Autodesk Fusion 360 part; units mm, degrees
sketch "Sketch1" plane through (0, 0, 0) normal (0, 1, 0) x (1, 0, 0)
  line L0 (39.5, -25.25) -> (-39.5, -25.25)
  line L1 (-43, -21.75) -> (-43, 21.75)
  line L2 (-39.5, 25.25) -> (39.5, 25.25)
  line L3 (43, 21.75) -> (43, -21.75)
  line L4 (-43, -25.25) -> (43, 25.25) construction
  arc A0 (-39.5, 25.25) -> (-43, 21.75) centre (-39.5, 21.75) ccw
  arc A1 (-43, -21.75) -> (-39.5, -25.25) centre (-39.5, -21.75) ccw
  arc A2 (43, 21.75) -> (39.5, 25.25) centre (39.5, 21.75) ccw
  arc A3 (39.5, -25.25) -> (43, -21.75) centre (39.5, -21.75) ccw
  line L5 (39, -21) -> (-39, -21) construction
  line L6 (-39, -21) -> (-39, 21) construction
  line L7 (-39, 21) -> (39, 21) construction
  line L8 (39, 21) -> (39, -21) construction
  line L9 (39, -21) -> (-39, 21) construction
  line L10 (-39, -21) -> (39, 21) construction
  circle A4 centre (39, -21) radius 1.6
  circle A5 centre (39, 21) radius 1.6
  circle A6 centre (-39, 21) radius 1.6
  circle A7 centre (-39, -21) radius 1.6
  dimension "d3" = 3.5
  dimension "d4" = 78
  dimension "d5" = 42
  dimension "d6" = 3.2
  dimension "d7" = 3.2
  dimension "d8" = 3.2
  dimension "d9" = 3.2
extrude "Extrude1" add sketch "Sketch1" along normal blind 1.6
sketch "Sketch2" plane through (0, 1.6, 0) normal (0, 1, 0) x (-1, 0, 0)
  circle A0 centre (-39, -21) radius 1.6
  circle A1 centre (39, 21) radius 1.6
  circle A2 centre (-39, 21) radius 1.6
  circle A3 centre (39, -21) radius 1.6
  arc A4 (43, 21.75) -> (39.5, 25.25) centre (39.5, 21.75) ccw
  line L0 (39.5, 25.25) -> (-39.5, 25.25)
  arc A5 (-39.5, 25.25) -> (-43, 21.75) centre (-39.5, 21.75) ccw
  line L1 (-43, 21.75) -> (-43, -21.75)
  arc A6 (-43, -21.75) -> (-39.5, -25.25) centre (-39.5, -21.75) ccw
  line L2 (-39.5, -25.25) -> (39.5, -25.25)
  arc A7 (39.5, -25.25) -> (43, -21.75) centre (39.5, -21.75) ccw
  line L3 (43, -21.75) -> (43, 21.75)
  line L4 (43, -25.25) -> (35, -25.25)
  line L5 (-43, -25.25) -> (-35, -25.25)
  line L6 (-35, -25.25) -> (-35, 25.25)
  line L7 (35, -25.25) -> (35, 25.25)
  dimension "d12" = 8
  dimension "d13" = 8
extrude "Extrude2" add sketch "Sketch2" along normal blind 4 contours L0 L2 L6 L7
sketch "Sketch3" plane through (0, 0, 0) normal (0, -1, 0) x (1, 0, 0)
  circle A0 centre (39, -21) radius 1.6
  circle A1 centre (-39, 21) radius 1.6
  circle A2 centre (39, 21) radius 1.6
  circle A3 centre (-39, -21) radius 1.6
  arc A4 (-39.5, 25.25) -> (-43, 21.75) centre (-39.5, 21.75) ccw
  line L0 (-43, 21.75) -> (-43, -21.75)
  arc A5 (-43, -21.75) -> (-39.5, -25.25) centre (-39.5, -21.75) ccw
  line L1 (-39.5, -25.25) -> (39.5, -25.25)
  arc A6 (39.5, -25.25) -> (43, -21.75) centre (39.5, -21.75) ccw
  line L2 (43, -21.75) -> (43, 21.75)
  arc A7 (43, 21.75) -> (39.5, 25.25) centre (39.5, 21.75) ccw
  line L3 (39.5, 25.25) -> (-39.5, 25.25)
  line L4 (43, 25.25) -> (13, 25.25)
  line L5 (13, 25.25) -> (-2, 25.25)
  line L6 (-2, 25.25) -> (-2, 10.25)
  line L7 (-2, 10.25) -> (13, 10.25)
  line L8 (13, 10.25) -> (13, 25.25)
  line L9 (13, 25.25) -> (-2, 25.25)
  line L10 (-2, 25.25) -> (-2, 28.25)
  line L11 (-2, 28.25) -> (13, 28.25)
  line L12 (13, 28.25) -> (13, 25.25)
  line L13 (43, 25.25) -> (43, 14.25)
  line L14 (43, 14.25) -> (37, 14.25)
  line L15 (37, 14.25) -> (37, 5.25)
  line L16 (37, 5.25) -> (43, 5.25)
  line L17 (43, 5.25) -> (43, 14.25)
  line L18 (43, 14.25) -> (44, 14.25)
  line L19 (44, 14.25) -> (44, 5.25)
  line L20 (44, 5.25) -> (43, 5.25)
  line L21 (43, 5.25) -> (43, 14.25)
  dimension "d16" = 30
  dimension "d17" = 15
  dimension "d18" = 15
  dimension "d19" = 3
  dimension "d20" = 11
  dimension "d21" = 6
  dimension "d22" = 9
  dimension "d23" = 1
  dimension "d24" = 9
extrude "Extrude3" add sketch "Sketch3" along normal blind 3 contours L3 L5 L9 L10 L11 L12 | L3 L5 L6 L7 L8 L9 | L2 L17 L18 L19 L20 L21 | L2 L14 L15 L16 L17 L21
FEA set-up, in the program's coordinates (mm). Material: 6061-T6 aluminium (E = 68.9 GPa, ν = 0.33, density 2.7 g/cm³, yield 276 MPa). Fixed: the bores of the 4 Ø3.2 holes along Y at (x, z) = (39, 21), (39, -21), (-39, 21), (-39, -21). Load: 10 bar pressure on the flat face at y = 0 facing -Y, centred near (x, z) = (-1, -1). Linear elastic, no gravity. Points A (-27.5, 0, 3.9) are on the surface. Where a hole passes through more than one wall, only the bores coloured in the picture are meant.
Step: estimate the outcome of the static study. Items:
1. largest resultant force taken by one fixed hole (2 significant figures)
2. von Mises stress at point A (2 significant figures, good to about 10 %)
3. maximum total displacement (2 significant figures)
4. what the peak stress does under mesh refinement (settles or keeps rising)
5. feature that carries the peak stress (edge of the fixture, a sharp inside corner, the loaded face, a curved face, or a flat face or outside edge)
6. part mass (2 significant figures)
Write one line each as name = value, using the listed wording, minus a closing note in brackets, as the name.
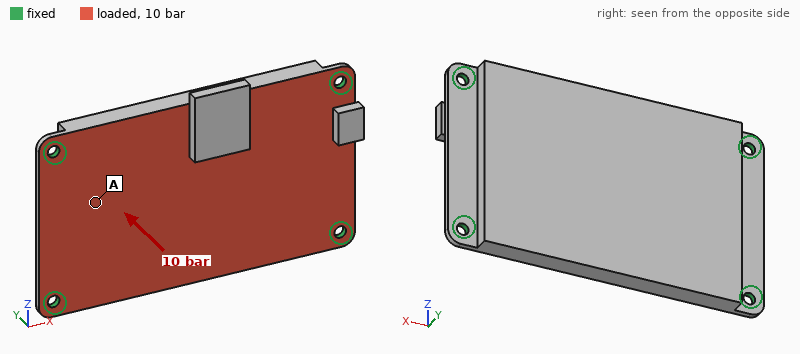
largest resultant force taken by one fixed hole = 2.3 kN
von Mises stress at point A = 28 MPa
maximum total displacement = 0.26 mm
what the peak stress does under mesh refinement = keeps rising
feature that carries the peak stress = edge of the fixture
part mass = 59 g
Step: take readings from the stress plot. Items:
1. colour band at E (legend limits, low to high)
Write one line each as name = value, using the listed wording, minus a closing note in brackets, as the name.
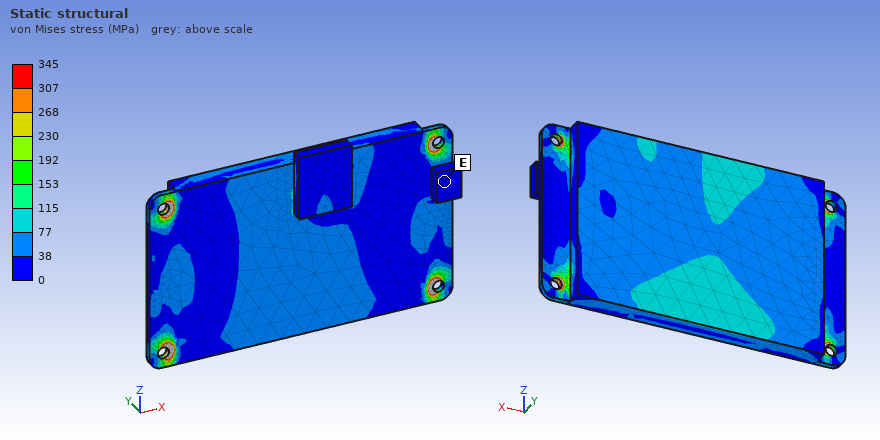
colour band at E = 0 to 38 MPa
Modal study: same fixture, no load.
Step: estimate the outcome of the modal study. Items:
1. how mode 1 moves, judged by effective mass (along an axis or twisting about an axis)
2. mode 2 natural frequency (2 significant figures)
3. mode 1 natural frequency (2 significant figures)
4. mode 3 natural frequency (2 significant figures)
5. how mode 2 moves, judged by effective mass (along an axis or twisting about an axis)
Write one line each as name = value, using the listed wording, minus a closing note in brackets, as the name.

how mode 1 moves, judged by effective mass = along Y
mode 2 natural frequency = 4600 Hz
mode 1 natural frequency = 2800 Hz
mode 3 natural frequency = 6800 Hz
how mode 2 moves, judged by effective mass = twisting about X
